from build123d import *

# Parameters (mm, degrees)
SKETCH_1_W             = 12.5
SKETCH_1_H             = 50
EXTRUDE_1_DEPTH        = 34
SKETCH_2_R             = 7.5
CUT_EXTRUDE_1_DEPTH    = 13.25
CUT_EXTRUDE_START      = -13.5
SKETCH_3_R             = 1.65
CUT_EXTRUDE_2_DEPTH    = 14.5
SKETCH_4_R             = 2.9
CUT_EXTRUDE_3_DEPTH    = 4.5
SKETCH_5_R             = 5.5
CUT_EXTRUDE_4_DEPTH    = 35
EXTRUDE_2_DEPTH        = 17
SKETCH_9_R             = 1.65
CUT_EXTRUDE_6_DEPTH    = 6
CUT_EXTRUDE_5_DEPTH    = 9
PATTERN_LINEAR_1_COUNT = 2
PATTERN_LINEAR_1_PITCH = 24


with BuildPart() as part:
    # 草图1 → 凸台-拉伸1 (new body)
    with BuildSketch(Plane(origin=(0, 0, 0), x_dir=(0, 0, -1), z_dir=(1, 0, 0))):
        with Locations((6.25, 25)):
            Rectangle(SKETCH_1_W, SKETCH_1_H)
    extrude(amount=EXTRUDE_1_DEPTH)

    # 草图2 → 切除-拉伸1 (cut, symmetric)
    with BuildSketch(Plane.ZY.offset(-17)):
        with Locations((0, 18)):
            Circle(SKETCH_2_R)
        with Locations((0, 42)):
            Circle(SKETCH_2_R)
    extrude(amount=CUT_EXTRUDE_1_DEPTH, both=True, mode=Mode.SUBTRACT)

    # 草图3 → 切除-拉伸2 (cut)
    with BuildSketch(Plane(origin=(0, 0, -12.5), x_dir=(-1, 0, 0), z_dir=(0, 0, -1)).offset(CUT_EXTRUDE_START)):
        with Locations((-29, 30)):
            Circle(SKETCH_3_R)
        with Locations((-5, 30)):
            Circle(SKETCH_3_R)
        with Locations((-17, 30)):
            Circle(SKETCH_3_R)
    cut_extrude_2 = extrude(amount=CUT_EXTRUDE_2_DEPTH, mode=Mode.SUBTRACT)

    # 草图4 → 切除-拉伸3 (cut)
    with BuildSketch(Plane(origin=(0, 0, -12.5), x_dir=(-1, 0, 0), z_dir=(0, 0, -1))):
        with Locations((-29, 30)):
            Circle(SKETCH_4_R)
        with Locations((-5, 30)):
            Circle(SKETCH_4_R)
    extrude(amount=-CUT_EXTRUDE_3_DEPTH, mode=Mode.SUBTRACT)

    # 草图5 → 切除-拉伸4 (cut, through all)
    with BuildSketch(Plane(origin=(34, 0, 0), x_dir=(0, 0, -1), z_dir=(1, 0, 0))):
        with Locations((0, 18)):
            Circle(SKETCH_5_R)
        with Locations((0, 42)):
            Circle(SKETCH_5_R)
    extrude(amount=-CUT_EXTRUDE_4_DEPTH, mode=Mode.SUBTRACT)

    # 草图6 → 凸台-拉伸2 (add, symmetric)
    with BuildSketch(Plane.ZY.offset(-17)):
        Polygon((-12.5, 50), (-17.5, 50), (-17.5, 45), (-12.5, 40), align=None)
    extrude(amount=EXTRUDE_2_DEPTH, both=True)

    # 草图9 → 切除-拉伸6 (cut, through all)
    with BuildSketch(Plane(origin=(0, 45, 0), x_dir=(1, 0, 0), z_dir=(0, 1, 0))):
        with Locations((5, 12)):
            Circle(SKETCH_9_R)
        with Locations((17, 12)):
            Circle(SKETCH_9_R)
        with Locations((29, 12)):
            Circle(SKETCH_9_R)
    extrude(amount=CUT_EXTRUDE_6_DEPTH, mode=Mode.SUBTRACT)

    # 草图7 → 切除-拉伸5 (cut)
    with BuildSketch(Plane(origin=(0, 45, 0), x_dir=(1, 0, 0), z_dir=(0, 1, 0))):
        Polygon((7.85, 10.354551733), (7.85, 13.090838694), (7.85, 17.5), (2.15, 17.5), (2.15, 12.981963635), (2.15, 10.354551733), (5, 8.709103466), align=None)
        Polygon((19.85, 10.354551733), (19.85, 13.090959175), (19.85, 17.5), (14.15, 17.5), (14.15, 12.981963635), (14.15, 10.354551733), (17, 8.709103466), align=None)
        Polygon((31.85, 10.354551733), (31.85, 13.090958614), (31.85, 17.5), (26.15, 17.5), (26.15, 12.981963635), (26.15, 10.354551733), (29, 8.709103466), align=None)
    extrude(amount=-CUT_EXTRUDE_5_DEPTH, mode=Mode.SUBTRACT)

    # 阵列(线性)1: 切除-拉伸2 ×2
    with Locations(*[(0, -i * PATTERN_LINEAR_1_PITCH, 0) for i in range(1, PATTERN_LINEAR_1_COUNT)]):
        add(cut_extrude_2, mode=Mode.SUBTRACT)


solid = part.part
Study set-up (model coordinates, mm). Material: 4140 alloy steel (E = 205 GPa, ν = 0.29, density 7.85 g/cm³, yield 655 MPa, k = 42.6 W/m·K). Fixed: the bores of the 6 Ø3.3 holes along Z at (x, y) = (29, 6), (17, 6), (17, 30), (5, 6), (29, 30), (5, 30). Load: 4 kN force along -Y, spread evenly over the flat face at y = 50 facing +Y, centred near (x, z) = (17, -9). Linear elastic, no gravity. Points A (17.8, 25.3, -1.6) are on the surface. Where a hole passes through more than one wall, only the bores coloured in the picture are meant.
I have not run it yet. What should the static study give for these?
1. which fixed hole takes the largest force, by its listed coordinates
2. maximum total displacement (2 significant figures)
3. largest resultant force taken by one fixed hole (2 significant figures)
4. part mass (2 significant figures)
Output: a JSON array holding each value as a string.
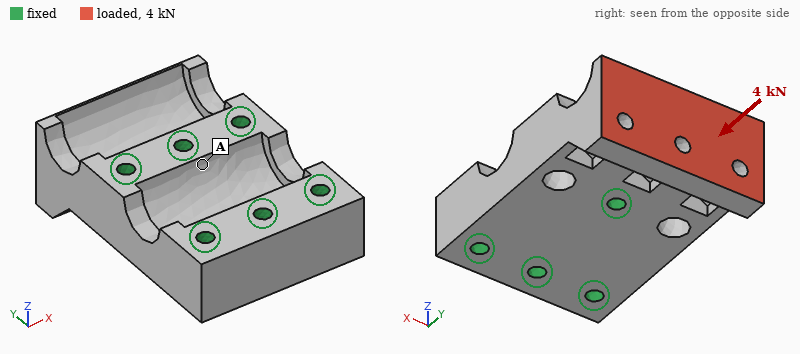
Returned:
["(17, 30)", "23 µm", "1.5 kN", "120 g"]
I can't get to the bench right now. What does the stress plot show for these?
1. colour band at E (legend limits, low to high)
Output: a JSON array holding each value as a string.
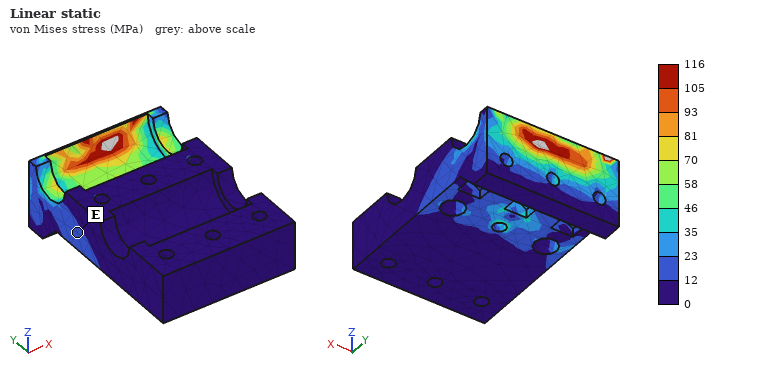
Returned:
["12 to 23 MPa"]
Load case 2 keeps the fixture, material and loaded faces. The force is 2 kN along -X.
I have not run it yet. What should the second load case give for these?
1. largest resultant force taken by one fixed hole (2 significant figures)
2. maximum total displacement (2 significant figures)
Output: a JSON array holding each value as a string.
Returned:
["1.3 kN", "9.1 µm"]
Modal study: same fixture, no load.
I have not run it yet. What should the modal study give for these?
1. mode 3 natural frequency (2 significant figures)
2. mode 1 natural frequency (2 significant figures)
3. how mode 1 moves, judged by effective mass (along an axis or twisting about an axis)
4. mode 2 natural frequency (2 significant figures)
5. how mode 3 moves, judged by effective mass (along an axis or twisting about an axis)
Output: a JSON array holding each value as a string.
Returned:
["22 kHz", "11 kHz", "along Z", "16 kHz", "along X"]
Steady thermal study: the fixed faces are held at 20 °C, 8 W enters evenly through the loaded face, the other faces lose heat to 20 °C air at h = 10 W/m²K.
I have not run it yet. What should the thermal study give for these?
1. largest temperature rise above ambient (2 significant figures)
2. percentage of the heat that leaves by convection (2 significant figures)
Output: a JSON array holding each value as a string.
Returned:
["22 K", "3.5 %"]
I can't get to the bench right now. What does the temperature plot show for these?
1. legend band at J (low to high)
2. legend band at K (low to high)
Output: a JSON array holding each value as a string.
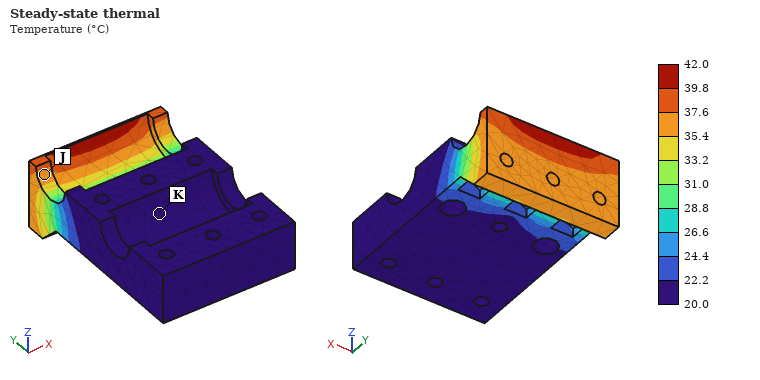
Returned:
["35.4 to 37.6 °C", "20.0 to 22.2 °C"]
